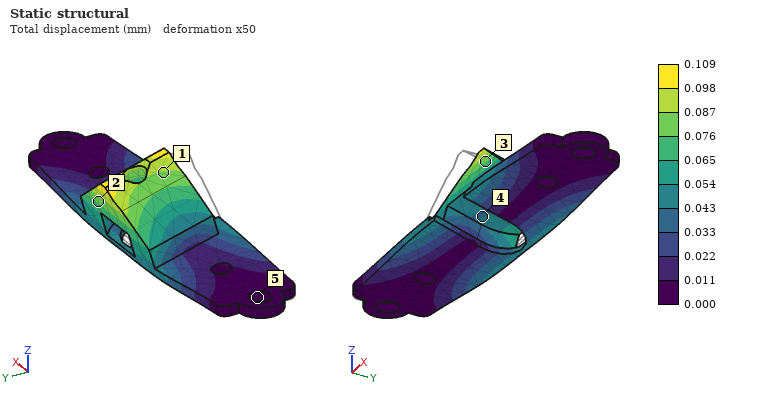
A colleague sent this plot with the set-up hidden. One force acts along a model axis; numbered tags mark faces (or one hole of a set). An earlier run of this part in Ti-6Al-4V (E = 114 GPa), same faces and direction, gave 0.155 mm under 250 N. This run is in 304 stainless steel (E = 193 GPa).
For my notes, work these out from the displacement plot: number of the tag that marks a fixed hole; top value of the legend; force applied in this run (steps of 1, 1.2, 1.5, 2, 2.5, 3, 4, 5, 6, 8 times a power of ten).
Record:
5
0.109 mm
300 N
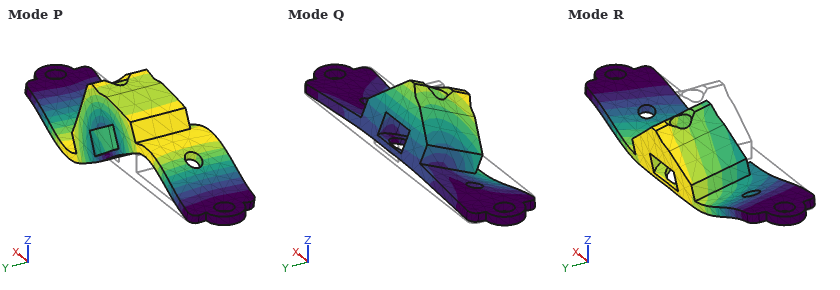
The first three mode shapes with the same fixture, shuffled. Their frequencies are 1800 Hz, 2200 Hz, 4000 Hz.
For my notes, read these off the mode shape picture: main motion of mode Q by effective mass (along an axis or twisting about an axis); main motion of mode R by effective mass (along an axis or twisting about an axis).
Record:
along Y
along Z
